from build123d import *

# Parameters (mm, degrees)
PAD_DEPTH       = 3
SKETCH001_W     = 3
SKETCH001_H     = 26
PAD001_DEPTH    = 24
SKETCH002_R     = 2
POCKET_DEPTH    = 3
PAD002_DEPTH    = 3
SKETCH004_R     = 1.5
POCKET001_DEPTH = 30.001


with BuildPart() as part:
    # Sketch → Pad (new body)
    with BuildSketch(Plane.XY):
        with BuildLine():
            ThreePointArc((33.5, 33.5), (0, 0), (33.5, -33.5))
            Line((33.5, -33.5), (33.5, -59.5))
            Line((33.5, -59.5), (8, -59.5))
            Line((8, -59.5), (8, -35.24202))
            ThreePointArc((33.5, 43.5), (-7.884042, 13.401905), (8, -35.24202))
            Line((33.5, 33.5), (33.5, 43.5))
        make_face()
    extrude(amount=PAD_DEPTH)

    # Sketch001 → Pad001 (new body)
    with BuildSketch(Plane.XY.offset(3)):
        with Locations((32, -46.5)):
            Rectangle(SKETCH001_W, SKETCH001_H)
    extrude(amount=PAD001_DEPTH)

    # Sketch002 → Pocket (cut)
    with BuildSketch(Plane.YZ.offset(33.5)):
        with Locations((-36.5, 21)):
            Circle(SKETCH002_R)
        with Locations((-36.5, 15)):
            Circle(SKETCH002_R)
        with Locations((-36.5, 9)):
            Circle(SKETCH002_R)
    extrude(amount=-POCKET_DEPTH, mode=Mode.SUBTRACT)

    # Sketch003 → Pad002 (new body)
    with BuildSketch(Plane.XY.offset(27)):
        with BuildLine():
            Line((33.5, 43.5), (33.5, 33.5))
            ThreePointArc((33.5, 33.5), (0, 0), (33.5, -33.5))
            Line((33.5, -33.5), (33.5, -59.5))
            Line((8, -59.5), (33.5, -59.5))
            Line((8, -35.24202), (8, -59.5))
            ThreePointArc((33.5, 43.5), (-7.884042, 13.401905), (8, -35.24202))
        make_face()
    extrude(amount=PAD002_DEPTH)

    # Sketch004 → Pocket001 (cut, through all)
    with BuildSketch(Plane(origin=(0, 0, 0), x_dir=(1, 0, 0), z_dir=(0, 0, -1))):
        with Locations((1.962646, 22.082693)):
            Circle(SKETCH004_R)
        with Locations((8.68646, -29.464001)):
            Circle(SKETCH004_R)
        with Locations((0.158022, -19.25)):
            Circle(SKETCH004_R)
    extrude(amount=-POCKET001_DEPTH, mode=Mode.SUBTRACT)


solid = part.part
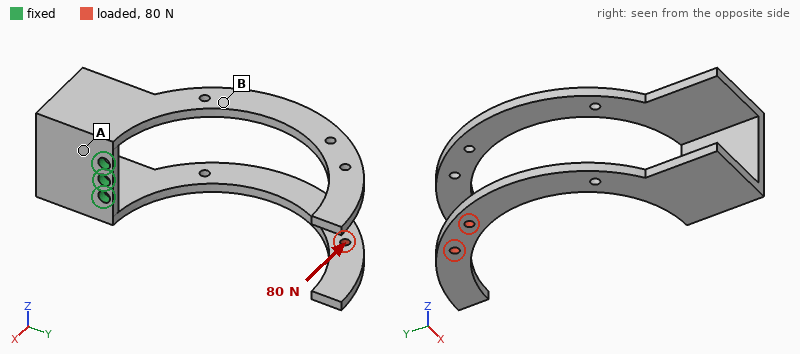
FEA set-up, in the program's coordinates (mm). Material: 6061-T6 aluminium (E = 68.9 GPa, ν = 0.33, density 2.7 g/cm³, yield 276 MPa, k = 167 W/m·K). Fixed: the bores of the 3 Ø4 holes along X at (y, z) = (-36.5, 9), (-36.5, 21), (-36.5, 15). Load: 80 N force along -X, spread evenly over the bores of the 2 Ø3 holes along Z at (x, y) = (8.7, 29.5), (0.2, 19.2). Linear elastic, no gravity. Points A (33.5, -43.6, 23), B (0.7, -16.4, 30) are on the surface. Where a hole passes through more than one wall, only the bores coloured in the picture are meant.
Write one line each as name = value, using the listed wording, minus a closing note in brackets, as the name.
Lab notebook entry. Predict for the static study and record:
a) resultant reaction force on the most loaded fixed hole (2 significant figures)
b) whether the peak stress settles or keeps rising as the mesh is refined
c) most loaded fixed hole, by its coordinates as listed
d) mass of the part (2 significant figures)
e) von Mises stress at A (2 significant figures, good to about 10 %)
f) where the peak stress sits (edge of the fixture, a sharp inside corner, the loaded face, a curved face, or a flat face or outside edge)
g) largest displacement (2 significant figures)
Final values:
resultant reaction force on the most loaded fixed hole = 100 N
whether the peak stress settles or keeps rising as the mesh is refined = keeps rising
most loaded fixed hole, by its coordinates as listed = (-36.5, 9)
mass of the part = 32 g
von Mises stress at A = 23 MPa
where the peak stress sits = edge of the fixture
largest displacement = 1.3 mm
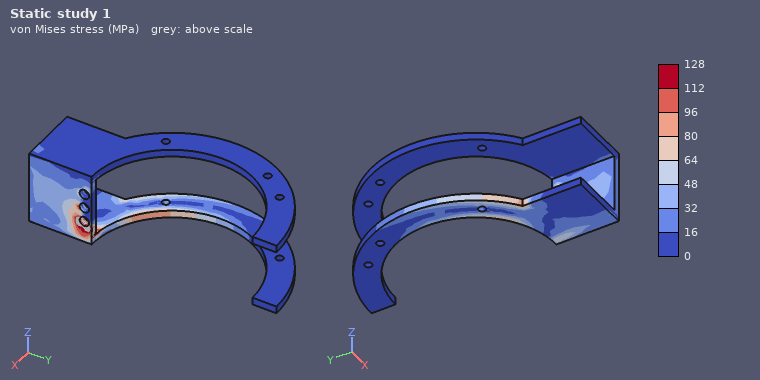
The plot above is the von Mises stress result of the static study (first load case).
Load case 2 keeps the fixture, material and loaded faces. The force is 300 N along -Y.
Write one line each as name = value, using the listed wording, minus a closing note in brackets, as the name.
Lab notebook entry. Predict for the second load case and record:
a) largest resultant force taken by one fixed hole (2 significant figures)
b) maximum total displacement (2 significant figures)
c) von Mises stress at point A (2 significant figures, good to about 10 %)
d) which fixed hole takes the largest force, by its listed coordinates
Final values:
largest resultant force taken by one fixed hole = 390 N
maximum total displacement = 0.88 mm
von Mises stress at point A = 42 MPa
which fixed hole takes the largest force, by its listed coordinates = (-36.5, 9)
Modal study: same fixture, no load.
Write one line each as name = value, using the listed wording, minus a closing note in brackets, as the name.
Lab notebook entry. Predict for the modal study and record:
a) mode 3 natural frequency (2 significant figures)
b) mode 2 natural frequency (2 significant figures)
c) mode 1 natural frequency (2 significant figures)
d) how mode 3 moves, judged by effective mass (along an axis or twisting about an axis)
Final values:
mode 3 natural frequency = 590 Hz
mode 2 natural frequency = 250 Hz
mode 1 natural frequency = 250 Hz
how mode 3 moves, judged by effective mass = along X
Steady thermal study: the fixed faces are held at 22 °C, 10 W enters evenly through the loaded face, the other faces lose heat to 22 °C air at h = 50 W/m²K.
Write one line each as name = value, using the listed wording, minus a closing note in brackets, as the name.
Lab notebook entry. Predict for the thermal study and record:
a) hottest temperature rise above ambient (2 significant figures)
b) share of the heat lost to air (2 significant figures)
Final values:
hottest temperature rise above ambient = 73 K
share of the heat lost to air = 69 %
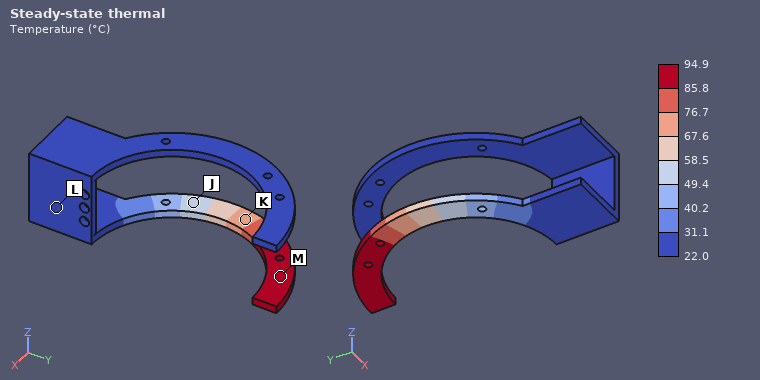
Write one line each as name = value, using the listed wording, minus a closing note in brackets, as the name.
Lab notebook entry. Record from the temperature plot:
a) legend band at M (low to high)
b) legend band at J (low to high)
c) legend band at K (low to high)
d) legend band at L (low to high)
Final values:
legend band at M = 85.8 to 94.9 °C
legend band at J = 49.4 to 58.5 °C
legend band at K = 67.6 to 76.7 °C
legend band at L = 22.0 to 31.1 °C
